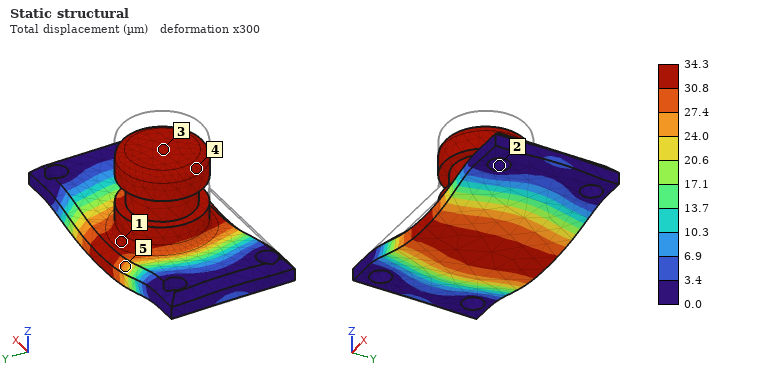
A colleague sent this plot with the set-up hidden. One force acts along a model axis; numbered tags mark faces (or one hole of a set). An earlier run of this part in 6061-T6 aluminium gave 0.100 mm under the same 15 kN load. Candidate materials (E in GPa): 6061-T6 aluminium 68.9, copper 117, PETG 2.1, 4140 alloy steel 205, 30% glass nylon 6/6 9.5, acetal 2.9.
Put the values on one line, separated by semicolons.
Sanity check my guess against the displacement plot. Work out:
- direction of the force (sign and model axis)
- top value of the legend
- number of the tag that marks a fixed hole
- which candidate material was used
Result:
-Z; 34.3 µm; 2; 4140 alloy steel
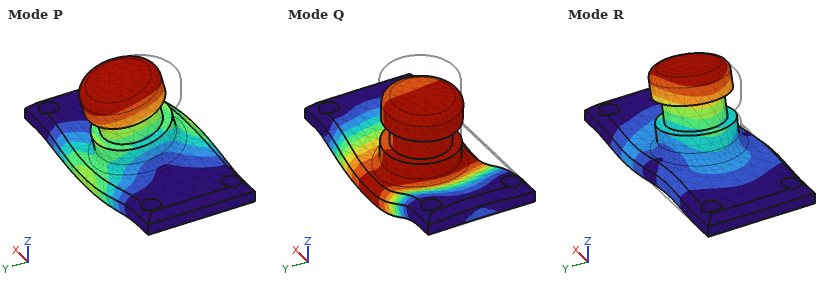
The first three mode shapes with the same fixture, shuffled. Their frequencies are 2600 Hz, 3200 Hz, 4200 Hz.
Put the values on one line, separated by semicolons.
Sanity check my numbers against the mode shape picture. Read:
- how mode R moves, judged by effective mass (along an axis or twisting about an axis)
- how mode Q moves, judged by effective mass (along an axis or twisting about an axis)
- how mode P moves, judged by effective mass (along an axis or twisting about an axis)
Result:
along X; along Z; along Y
